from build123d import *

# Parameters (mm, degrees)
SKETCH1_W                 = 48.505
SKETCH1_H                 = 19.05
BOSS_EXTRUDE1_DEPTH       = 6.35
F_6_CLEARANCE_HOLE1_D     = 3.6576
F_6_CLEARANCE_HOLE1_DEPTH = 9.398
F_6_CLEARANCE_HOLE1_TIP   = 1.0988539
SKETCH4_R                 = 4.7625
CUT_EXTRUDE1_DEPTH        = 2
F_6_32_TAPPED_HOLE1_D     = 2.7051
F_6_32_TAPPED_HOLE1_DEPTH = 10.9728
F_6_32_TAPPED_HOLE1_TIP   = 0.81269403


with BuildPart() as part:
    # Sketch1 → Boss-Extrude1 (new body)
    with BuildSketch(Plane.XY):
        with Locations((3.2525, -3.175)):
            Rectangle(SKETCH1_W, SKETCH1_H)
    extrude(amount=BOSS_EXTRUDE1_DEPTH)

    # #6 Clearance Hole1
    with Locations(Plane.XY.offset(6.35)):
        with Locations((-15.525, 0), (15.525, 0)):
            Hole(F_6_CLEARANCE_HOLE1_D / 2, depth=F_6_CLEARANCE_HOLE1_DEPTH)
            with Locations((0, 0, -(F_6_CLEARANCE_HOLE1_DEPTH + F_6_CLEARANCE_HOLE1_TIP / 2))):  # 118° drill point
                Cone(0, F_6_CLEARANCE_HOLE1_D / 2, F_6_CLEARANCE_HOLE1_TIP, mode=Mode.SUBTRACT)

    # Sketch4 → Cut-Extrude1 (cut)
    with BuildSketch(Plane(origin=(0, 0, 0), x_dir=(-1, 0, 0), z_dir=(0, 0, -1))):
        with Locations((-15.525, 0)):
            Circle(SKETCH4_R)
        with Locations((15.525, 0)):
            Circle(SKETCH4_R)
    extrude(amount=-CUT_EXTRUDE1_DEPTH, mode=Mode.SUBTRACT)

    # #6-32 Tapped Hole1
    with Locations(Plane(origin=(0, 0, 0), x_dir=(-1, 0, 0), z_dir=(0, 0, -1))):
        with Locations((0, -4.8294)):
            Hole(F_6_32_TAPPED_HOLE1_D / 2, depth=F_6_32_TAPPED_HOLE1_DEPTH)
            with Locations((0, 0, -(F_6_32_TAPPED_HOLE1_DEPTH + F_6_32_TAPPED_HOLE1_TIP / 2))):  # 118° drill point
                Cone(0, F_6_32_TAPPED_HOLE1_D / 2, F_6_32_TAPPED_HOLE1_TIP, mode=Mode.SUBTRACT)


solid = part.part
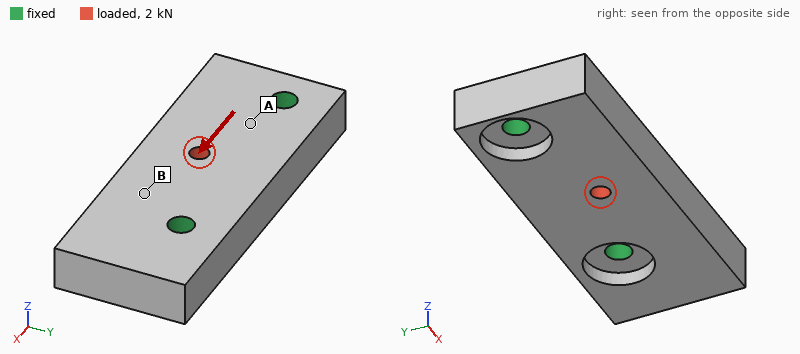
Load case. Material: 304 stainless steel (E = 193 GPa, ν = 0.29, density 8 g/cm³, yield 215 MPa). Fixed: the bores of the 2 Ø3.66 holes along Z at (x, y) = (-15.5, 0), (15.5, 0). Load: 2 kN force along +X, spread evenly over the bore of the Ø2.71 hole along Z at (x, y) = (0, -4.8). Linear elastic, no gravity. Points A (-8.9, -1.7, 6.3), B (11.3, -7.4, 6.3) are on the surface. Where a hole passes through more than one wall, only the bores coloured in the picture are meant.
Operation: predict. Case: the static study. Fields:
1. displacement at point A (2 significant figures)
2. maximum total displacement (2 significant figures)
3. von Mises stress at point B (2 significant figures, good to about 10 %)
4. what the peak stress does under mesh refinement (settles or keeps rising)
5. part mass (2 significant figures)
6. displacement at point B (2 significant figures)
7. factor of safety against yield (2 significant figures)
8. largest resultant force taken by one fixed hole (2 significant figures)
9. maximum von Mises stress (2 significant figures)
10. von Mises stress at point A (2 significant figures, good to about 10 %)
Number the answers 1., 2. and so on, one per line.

1. 0.64 µm
2. 1.9 µm
3. 9.2 MPa
4. settles
5. 44 g
6. 0.91 µm
7. 3.3
8. 1.1 kN
9. 65 MPa
10. 22 MPa
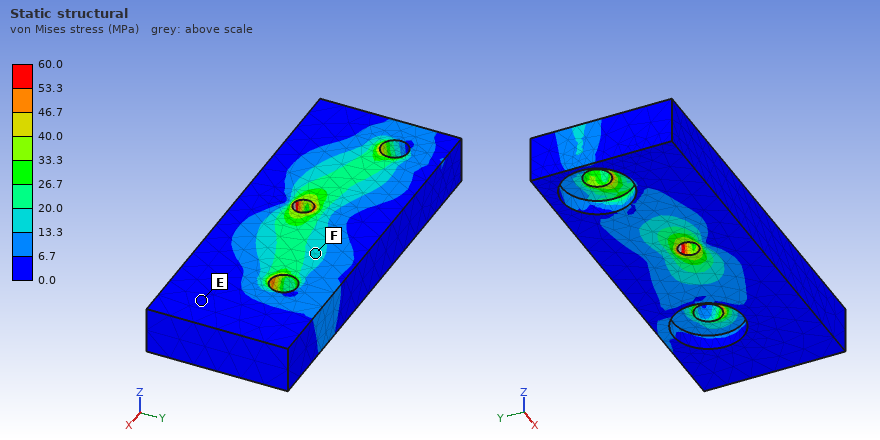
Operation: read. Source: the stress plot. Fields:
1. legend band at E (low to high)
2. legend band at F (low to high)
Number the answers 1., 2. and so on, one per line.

1. 0.0 to 6.7 MPa
2. 13.3 to 20.0 MPa
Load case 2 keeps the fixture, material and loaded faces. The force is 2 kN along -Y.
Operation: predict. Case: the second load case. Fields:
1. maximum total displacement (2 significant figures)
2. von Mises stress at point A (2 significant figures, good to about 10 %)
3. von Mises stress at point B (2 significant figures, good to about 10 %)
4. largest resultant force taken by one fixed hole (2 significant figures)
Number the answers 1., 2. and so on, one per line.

1. 4.5 µm
2. 19 MPa
3. 16 MPa
4. 1.1 kN
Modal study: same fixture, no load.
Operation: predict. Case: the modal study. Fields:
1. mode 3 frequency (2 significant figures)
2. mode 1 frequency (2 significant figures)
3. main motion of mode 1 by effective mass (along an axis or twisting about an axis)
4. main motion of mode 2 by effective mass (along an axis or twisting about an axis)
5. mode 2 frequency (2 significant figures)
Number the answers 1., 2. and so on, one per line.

1. 23 kHz
2. 14 kHz
3. along Z
4. twisting about Y
5. 17 kHz
